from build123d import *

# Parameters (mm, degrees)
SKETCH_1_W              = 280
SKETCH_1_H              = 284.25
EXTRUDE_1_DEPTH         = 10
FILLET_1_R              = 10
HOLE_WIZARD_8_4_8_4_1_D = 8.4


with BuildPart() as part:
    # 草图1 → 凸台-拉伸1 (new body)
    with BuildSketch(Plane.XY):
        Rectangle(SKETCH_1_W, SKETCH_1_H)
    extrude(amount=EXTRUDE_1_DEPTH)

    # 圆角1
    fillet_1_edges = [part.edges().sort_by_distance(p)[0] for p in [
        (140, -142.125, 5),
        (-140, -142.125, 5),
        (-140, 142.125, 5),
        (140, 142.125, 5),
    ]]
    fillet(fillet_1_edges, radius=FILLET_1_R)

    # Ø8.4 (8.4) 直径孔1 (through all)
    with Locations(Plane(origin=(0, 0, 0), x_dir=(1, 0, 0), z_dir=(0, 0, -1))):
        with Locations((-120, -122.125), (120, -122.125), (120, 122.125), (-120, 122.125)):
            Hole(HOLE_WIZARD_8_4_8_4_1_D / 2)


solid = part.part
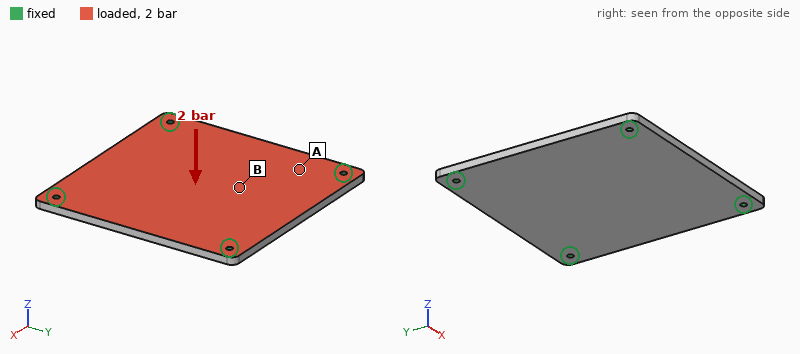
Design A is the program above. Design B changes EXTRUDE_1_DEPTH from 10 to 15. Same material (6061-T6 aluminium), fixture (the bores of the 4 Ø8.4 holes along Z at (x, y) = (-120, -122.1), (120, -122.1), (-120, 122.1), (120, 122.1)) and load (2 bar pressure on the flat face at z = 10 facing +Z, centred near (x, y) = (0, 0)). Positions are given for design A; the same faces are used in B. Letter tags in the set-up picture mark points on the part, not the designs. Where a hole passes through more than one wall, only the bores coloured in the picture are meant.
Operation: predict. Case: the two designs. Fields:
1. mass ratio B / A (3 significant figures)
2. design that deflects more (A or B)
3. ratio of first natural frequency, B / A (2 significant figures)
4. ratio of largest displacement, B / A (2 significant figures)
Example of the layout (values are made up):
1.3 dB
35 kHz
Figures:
1.50
A
1.4
0.32
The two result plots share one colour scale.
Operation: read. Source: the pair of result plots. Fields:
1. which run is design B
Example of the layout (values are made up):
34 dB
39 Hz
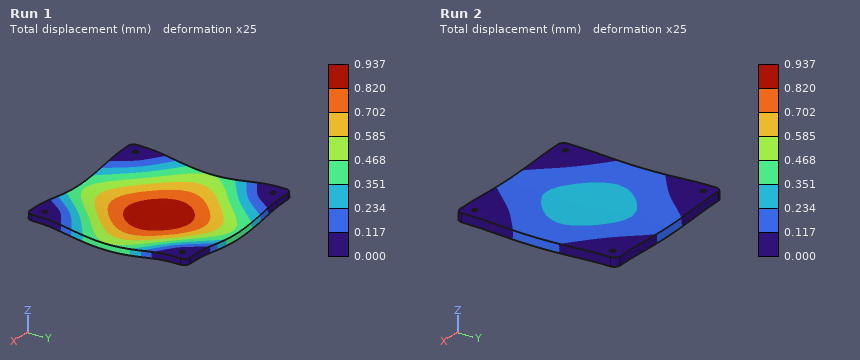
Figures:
Run 2
